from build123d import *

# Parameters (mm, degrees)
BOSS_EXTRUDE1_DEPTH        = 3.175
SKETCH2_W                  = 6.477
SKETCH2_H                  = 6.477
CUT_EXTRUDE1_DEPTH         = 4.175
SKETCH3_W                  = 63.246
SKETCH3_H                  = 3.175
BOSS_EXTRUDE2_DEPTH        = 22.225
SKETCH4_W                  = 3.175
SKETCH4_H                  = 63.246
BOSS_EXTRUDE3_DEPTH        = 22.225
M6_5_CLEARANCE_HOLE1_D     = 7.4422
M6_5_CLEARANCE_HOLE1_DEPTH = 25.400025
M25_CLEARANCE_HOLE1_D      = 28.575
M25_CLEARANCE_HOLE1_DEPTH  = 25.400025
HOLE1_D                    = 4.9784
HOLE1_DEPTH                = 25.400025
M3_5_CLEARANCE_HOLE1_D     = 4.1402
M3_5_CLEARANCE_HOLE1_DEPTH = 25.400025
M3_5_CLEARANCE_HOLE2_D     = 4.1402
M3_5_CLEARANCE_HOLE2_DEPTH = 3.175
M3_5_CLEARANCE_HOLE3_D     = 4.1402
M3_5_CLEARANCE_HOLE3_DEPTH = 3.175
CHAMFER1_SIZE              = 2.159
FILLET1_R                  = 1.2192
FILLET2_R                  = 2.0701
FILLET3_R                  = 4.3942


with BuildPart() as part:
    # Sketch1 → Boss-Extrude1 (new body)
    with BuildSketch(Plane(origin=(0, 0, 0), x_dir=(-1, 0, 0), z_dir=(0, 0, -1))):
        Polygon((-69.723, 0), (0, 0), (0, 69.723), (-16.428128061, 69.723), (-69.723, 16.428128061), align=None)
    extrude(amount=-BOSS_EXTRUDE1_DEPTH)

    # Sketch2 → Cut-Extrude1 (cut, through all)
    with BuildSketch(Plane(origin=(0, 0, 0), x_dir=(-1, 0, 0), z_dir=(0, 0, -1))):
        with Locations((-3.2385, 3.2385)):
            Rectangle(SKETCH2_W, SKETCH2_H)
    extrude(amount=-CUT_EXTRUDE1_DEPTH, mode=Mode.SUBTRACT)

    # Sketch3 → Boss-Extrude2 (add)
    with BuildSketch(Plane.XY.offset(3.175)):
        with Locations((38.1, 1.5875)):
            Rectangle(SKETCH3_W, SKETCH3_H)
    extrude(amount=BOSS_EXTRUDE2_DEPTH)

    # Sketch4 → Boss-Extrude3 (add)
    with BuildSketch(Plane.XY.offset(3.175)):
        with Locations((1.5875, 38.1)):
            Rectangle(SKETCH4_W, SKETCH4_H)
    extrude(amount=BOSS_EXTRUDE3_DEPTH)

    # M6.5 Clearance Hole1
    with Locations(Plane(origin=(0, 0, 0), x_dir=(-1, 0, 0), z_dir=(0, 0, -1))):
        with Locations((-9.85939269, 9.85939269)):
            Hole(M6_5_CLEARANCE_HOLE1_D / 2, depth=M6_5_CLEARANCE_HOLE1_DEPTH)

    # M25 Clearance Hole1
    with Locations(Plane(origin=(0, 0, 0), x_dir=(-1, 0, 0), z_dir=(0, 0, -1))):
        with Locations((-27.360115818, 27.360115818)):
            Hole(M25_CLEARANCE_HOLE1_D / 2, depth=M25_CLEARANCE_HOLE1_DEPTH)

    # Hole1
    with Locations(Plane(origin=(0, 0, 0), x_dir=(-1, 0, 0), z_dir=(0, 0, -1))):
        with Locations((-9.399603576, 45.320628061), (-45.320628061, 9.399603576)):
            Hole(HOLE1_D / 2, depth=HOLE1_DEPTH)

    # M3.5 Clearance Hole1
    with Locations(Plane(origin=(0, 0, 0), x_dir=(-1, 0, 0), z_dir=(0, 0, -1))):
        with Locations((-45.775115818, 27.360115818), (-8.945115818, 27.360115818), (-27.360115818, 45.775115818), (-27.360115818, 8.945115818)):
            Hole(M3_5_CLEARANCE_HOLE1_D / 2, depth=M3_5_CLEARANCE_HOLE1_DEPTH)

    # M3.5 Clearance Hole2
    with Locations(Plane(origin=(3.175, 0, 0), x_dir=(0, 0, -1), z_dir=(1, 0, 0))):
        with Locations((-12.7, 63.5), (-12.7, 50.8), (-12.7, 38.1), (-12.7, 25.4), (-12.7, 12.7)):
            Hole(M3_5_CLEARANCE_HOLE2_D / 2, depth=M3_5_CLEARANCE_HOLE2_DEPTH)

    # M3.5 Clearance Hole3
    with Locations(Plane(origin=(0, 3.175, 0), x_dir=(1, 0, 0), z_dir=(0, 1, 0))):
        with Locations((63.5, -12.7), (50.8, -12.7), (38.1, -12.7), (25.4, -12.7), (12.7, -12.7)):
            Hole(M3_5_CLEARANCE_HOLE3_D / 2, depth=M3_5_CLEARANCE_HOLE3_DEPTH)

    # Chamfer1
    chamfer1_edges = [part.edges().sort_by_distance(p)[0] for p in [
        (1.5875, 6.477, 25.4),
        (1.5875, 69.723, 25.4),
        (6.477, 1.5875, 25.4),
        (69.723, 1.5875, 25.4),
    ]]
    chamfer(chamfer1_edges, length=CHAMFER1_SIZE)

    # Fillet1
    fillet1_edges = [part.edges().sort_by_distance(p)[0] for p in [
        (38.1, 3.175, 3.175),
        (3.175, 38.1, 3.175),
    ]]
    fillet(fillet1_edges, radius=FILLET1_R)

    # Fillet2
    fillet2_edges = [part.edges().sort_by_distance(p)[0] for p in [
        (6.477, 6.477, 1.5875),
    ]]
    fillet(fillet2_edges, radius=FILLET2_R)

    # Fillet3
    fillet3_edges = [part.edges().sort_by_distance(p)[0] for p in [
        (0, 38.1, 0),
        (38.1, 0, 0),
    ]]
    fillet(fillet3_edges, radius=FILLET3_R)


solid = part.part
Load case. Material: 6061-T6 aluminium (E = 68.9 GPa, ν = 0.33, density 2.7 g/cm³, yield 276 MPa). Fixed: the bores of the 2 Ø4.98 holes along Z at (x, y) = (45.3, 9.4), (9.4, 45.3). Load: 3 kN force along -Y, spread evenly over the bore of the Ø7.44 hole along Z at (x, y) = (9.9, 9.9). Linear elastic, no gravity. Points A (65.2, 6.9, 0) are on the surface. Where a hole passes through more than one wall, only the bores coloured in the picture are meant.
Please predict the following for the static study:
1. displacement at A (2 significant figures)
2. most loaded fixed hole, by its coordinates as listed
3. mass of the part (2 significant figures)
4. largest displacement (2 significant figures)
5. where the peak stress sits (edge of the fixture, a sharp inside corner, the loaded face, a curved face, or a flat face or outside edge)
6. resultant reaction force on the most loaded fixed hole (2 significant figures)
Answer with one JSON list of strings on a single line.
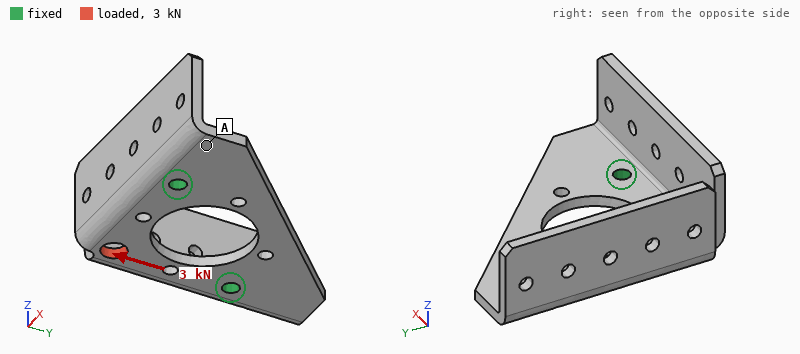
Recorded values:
["10.0 µm", "(9.4, 45.3)", "44 g", "48 µm", "a curved face", "2.6 kN"]
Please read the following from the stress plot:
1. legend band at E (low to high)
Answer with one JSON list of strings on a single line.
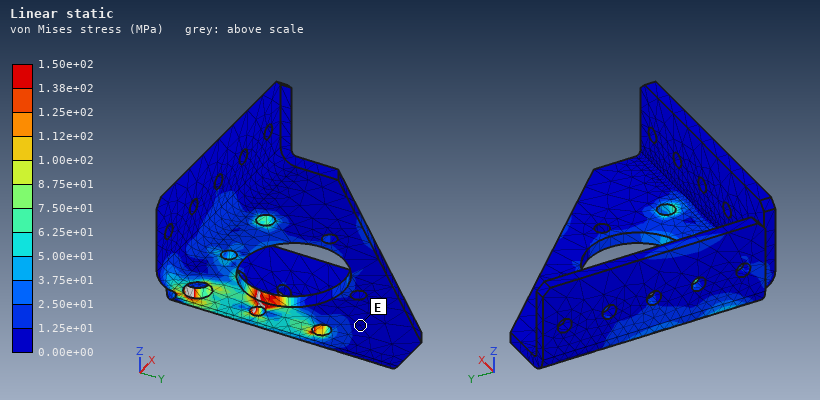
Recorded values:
["0.00e+00 to 1.25e+01 MPa"]
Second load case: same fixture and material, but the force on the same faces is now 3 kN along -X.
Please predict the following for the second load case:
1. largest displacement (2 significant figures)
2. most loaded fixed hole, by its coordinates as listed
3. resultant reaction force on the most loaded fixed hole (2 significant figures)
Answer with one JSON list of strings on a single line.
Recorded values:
["48 µm", "(45.3, 9.4)", "2.6 kN"]
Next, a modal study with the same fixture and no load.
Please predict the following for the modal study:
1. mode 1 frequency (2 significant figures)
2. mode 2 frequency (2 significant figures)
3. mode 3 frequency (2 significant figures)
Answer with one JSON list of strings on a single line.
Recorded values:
["2000 Hz", "2700 Hz", "2700 Hz"]
